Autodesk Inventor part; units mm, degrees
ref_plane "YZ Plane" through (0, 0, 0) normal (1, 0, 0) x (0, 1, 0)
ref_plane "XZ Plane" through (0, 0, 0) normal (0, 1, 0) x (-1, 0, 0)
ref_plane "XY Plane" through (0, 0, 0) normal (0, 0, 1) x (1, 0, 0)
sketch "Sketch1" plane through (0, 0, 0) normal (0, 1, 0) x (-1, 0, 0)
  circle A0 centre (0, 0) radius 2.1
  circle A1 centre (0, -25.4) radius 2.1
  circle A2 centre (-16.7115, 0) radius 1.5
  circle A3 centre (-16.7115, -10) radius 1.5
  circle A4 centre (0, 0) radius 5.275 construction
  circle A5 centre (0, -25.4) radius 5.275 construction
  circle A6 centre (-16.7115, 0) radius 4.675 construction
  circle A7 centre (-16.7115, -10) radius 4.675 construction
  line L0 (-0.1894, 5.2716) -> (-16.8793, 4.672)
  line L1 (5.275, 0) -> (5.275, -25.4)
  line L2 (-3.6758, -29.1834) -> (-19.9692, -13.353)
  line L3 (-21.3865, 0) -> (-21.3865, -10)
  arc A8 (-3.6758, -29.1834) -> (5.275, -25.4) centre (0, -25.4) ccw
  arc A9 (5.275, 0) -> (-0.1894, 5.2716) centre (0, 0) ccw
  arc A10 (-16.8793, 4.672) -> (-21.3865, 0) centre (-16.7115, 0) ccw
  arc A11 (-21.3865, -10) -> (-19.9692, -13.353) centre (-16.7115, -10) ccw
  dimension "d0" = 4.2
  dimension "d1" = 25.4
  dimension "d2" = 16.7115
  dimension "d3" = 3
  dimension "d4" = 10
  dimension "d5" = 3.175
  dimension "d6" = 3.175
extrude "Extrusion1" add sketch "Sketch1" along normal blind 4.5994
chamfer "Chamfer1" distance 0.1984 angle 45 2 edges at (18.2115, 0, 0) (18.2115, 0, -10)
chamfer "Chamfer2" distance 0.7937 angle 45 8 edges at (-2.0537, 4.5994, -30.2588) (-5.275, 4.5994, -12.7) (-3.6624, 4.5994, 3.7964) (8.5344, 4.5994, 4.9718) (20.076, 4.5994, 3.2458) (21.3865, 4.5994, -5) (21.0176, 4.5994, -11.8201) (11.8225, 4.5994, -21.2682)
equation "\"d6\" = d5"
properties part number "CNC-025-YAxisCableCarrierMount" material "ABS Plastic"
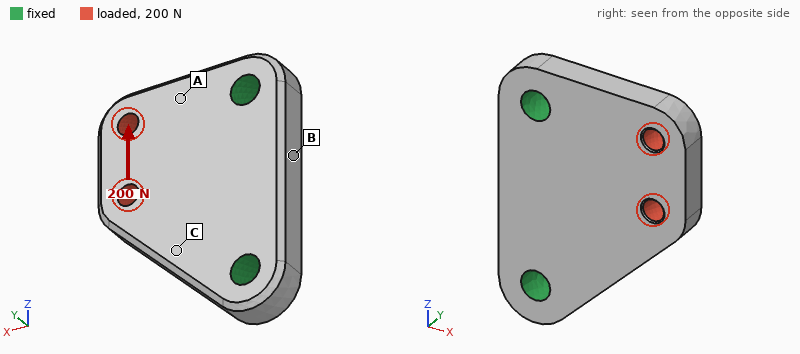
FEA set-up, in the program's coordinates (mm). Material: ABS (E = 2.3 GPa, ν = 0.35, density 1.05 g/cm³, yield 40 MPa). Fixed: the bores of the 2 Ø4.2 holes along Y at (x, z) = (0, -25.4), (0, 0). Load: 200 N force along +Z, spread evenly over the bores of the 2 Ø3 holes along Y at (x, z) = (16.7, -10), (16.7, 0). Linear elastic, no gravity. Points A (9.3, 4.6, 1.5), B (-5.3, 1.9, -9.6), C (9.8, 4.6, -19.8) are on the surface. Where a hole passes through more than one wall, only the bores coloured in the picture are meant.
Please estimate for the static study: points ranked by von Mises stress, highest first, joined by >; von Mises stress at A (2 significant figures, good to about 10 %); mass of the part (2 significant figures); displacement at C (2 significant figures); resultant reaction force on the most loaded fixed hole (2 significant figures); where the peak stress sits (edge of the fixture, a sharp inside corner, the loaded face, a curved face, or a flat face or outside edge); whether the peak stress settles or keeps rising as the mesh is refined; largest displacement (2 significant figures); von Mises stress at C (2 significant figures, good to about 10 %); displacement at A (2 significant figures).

C > A > B
2.3 MPa
3.4 g
19 µm
160 N
edge of the fixture
keeps rising
63 µm
3.9 MPa
26 µm
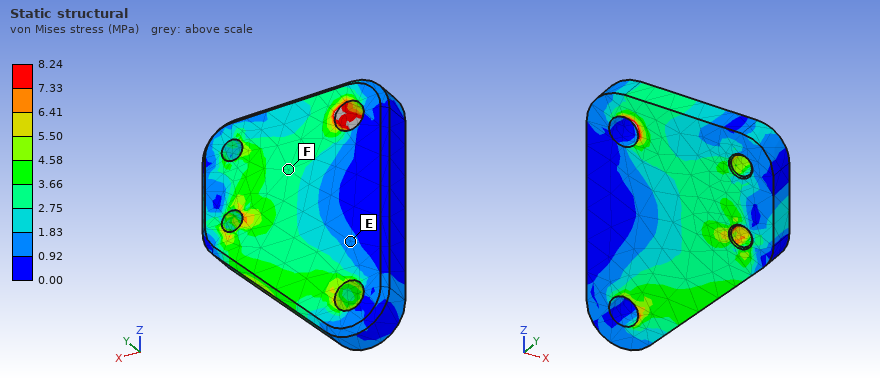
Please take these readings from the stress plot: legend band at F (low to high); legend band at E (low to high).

2.75 to 3.66 MPa
0.92 to 1.83 MPa
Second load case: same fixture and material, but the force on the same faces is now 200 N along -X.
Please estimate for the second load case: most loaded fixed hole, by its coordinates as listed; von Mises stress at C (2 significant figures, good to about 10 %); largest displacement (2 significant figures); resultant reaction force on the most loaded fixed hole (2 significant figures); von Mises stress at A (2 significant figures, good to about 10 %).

(0, 0)
1.0 MPa
27 µm
160 N
3.0 MPa
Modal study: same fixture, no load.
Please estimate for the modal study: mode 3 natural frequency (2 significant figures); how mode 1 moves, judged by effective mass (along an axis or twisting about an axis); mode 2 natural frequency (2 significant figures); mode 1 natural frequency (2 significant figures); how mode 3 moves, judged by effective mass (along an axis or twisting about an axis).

10000 Hz
along Y
6200 Hz
2700 Hz
along Z
